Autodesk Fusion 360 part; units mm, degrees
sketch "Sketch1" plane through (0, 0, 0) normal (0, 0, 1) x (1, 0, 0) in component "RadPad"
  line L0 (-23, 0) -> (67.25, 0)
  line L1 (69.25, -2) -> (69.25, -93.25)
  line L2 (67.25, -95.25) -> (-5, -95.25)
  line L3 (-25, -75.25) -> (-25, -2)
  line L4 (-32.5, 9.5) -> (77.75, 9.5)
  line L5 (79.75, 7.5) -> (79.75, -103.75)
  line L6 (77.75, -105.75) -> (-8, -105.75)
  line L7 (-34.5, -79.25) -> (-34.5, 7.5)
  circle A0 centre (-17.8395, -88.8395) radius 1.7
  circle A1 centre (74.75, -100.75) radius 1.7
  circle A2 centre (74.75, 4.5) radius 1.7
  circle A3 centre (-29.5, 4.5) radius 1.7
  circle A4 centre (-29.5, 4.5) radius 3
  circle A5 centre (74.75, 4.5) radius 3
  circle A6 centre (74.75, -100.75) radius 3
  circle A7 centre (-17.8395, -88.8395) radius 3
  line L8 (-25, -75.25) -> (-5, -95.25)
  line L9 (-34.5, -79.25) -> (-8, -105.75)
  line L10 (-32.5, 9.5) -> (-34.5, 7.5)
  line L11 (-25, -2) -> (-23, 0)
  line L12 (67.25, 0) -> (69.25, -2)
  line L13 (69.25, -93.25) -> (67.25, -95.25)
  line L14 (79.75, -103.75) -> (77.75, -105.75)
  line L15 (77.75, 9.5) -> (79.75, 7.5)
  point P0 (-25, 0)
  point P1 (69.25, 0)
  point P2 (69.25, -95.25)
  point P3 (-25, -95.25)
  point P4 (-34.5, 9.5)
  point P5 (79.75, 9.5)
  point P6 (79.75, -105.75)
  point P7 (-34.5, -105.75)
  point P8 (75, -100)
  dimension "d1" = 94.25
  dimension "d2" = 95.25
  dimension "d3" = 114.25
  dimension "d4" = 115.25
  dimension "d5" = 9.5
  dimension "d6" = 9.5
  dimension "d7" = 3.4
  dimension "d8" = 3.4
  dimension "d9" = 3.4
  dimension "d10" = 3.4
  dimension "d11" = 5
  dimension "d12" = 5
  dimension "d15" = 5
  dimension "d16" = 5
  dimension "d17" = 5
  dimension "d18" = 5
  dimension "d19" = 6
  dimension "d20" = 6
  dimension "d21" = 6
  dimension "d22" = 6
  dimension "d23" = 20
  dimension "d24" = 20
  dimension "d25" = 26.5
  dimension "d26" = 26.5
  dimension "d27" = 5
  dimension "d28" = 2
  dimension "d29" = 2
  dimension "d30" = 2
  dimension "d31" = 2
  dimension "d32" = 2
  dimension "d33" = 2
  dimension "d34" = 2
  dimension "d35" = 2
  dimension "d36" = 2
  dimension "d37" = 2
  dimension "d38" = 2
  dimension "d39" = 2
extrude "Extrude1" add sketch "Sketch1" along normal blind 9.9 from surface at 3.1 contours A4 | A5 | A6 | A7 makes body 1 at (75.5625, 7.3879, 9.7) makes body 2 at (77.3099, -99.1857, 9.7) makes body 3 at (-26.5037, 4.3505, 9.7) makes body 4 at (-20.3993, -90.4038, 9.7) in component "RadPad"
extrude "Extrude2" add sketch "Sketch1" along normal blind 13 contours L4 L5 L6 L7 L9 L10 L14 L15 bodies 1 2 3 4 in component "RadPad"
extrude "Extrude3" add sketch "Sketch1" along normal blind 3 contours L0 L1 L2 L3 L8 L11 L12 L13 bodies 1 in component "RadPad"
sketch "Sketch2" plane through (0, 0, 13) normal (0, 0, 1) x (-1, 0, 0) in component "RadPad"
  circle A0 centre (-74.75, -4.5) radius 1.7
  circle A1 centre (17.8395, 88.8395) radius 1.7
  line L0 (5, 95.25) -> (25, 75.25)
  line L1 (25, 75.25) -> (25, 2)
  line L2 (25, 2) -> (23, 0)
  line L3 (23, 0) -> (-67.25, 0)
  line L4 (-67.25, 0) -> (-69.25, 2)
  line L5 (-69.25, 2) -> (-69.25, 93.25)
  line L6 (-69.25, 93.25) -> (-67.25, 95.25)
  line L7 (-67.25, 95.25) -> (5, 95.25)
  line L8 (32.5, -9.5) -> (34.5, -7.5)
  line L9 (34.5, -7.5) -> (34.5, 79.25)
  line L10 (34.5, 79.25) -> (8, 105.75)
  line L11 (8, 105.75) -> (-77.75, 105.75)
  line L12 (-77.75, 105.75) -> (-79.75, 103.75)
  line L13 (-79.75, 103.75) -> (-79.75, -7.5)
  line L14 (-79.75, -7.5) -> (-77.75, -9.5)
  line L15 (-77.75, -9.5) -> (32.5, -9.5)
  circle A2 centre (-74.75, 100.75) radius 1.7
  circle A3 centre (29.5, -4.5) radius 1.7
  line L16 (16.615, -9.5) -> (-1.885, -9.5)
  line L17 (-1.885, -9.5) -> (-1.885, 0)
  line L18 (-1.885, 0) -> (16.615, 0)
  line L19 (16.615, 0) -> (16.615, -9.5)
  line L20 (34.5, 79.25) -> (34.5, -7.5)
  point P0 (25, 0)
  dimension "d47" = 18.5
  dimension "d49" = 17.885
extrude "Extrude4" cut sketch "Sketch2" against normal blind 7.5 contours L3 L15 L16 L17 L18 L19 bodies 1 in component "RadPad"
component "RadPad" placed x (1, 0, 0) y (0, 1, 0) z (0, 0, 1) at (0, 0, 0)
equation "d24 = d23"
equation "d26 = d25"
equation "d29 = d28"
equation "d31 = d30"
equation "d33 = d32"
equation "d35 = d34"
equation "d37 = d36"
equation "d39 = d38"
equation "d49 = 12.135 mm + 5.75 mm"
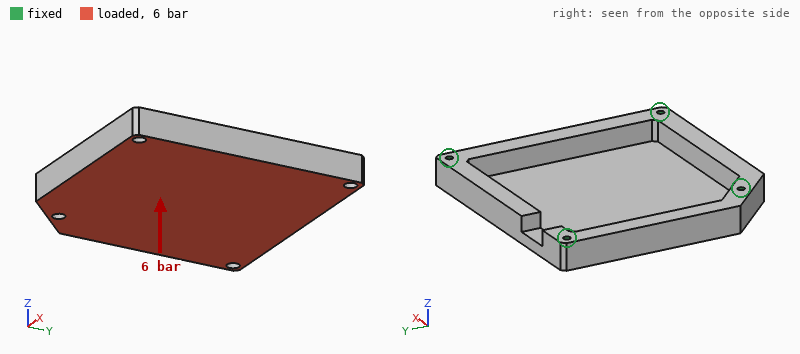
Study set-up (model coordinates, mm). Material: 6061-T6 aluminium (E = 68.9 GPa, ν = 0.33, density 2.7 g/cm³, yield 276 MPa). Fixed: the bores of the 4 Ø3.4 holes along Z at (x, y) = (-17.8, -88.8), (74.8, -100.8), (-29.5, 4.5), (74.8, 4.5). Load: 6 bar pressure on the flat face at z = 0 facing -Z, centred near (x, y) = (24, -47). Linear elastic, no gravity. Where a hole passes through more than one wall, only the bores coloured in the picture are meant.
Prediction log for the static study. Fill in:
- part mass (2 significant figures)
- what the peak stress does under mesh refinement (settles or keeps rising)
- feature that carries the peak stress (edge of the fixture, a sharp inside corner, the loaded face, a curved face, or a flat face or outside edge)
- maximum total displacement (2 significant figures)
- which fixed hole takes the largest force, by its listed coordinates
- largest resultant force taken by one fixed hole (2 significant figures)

210 g
keeps rising
edge of the fixture
0.57 mm
(74.8, 4.5)
3.0 kN
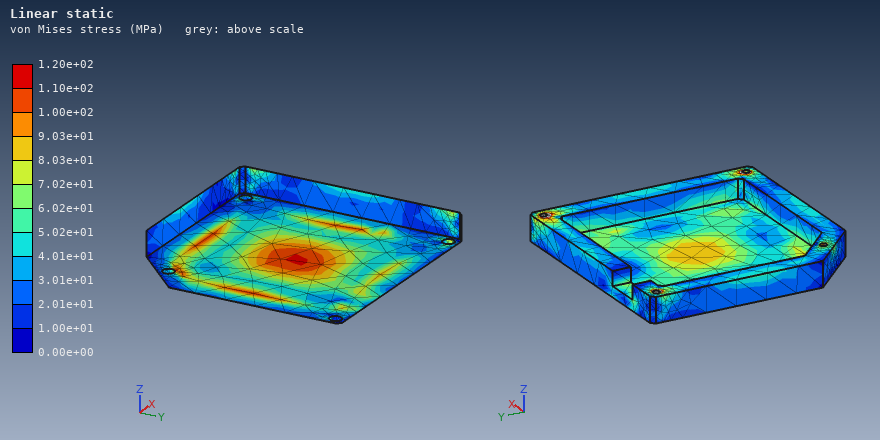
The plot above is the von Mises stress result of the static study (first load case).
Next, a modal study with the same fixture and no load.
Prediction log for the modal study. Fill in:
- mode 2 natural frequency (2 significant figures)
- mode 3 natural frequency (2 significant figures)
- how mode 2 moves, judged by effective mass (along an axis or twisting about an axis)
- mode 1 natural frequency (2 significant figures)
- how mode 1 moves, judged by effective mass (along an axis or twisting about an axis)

3900 Hz
4300 Hz
twisting about X
2300 Hz
along Z
